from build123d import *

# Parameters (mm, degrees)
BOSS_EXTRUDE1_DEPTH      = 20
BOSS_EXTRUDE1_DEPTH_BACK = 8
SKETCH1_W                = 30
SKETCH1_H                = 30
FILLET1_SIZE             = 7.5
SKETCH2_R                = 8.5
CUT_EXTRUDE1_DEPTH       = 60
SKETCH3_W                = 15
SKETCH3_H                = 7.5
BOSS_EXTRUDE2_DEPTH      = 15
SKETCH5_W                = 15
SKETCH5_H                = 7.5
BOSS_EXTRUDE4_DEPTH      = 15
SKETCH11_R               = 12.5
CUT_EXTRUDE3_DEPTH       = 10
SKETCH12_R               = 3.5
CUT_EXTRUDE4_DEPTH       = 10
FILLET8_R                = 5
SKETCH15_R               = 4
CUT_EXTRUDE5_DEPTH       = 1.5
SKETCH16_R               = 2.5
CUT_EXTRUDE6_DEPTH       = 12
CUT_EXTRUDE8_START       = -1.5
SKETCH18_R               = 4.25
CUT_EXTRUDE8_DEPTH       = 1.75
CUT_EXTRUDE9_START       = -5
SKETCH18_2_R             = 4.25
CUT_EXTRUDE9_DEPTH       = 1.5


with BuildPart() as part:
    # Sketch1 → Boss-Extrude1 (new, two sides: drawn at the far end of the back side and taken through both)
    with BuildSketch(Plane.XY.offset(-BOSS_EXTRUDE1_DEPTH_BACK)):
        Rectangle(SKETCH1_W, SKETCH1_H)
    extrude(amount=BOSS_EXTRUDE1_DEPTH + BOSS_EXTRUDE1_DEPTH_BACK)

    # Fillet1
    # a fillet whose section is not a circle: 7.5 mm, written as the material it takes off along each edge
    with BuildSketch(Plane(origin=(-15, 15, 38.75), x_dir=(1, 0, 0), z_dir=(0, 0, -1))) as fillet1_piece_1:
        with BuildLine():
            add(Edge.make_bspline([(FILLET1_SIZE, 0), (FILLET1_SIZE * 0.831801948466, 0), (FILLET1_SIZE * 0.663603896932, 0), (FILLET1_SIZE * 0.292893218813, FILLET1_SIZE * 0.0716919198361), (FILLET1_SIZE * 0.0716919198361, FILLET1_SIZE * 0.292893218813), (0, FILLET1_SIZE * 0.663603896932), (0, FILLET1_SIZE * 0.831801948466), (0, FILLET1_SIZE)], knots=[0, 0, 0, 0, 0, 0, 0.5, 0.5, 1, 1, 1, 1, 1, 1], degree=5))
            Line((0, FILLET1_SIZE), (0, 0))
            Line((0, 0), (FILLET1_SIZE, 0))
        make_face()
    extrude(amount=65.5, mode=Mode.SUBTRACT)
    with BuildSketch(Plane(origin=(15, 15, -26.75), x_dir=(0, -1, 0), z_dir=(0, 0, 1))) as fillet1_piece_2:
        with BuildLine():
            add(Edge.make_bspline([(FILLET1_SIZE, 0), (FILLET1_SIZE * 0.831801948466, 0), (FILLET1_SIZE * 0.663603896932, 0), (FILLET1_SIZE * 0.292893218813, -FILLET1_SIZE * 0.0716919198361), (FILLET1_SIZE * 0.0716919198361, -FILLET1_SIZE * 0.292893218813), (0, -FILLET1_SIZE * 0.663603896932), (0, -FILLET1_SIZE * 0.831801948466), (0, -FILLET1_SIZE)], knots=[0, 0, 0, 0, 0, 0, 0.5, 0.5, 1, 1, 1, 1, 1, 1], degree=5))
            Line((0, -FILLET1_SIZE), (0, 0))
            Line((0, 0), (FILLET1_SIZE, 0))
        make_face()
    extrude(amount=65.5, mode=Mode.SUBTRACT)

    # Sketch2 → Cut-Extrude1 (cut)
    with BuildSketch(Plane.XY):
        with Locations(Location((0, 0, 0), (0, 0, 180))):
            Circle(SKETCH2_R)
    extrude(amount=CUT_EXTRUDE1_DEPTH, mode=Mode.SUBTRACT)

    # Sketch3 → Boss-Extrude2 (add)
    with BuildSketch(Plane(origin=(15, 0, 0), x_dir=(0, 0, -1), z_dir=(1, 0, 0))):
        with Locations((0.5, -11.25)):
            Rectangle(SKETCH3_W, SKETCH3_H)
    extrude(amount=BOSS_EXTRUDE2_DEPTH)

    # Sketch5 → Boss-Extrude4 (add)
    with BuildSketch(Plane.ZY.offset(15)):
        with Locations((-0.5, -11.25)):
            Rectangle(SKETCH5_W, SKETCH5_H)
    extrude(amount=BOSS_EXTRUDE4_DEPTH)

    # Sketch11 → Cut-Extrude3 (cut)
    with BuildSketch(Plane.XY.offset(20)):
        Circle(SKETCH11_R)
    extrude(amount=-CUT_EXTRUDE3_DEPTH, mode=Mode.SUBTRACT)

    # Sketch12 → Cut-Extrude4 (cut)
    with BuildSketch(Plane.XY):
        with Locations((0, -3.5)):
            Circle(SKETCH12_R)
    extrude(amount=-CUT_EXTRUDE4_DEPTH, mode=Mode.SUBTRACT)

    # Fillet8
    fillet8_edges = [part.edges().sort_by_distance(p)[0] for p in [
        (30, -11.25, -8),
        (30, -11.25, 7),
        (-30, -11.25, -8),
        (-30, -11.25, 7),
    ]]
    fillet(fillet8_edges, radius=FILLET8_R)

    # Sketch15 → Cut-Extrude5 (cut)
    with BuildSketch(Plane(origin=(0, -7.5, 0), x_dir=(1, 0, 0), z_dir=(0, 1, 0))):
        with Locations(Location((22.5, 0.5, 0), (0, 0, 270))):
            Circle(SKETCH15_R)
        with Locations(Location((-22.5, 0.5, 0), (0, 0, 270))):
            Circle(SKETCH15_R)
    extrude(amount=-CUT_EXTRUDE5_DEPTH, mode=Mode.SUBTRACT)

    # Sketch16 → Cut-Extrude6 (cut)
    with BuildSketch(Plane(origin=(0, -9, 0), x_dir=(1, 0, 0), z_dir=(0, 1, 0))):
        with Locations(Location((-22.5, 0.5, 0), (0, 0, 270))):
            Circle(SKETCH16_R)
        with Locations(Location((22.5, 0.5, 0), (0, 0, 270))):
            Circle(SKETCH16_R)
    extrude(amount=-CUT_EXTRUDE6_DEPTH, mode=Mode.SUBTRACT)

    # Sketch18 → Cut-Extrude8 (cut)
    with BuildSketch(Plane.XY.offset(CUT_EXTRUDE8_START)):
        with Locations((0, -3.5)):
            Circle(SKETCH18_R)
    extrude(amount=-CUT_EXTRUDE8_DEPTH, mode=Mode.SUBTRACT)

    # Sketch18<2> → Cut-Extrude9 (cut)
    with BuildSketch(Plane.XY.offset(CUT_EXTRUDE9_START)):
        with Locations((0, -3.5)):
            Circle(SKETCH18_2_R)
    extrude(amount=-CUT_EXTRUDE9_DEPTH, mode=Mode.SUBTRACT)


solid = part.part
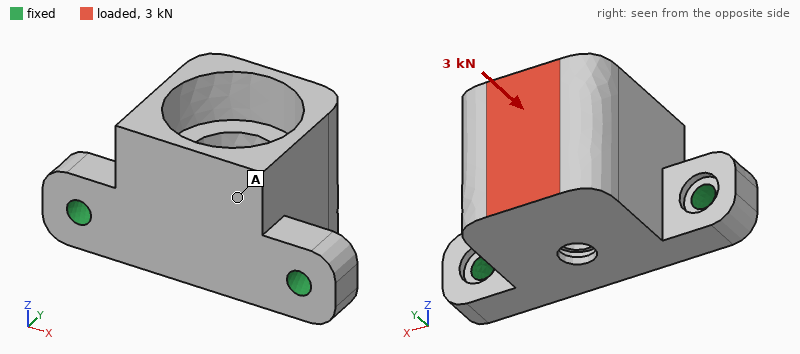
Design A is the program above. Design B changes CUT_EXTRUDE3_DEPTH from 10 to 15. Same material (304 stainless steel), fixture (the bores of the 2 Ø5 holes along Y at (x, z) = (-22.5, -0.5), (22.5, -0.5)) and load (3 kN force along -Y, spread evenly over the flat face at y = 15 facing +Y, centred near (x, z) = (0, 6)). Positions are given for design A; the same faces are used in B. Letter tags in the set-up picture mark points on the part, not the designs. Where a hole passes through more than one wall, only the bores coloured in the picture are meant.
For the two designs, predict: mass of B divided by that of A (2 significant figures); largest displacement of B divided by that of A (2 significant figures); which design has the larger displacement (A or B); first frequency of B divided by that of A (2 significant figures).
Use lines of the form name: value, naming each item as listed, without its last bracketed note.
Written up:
mass of B divided by that of A: 0.93
largest displacement of B divided by that of A: 1.1
which design has the larger displacement: B
first frequency of B divided by that of A: 1.0
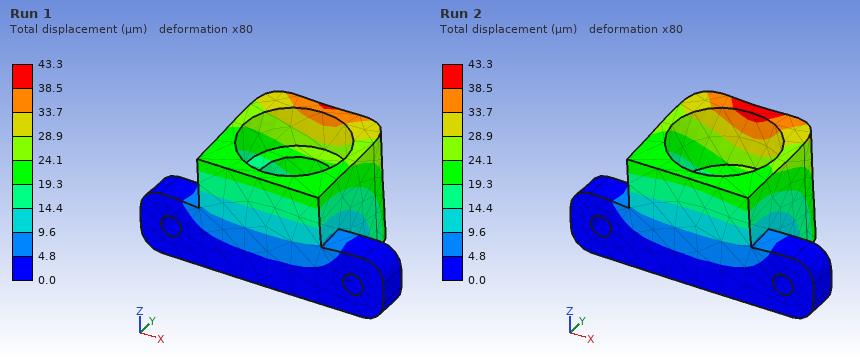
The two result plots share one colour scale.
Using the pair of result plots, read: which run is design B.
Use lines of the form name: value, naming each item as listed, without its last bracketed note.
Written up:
which run is design B: Run 2
